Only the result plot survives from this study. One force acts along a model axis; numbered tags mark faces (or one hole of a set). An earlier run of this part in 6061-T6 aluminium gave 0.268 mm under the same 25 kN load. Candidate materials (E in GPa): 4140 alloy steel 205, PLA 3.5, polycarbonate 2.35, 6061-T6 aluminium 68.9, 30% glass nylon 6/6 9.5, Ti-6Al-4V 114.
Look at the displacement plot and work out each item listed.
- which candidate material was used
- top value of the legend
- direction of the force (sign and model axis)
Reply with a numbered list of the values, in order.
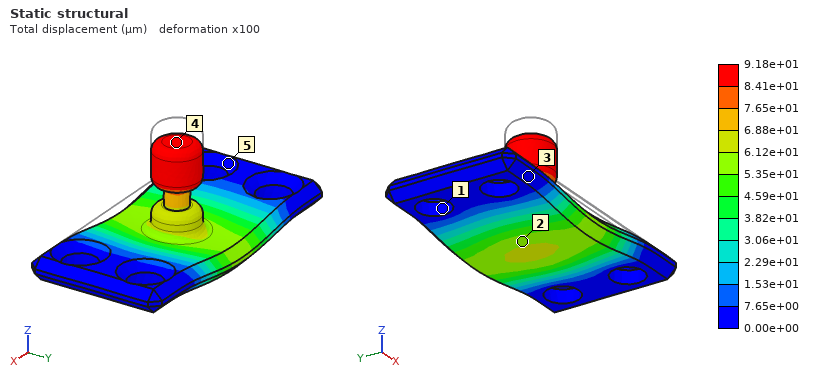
1. 4140 alloy steel
2. 9.18e+01 µm
3. -Z
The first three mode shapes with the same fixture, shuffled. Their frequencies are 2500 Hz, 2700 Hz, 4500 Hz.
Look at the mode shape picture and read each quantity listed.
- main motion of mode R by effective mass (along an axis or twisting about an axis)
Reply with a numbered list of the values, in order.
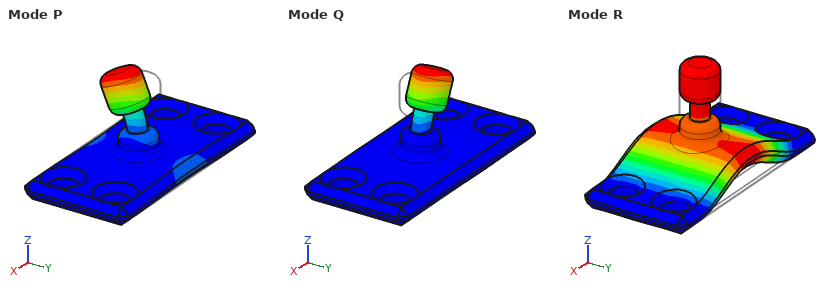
1. along Z
